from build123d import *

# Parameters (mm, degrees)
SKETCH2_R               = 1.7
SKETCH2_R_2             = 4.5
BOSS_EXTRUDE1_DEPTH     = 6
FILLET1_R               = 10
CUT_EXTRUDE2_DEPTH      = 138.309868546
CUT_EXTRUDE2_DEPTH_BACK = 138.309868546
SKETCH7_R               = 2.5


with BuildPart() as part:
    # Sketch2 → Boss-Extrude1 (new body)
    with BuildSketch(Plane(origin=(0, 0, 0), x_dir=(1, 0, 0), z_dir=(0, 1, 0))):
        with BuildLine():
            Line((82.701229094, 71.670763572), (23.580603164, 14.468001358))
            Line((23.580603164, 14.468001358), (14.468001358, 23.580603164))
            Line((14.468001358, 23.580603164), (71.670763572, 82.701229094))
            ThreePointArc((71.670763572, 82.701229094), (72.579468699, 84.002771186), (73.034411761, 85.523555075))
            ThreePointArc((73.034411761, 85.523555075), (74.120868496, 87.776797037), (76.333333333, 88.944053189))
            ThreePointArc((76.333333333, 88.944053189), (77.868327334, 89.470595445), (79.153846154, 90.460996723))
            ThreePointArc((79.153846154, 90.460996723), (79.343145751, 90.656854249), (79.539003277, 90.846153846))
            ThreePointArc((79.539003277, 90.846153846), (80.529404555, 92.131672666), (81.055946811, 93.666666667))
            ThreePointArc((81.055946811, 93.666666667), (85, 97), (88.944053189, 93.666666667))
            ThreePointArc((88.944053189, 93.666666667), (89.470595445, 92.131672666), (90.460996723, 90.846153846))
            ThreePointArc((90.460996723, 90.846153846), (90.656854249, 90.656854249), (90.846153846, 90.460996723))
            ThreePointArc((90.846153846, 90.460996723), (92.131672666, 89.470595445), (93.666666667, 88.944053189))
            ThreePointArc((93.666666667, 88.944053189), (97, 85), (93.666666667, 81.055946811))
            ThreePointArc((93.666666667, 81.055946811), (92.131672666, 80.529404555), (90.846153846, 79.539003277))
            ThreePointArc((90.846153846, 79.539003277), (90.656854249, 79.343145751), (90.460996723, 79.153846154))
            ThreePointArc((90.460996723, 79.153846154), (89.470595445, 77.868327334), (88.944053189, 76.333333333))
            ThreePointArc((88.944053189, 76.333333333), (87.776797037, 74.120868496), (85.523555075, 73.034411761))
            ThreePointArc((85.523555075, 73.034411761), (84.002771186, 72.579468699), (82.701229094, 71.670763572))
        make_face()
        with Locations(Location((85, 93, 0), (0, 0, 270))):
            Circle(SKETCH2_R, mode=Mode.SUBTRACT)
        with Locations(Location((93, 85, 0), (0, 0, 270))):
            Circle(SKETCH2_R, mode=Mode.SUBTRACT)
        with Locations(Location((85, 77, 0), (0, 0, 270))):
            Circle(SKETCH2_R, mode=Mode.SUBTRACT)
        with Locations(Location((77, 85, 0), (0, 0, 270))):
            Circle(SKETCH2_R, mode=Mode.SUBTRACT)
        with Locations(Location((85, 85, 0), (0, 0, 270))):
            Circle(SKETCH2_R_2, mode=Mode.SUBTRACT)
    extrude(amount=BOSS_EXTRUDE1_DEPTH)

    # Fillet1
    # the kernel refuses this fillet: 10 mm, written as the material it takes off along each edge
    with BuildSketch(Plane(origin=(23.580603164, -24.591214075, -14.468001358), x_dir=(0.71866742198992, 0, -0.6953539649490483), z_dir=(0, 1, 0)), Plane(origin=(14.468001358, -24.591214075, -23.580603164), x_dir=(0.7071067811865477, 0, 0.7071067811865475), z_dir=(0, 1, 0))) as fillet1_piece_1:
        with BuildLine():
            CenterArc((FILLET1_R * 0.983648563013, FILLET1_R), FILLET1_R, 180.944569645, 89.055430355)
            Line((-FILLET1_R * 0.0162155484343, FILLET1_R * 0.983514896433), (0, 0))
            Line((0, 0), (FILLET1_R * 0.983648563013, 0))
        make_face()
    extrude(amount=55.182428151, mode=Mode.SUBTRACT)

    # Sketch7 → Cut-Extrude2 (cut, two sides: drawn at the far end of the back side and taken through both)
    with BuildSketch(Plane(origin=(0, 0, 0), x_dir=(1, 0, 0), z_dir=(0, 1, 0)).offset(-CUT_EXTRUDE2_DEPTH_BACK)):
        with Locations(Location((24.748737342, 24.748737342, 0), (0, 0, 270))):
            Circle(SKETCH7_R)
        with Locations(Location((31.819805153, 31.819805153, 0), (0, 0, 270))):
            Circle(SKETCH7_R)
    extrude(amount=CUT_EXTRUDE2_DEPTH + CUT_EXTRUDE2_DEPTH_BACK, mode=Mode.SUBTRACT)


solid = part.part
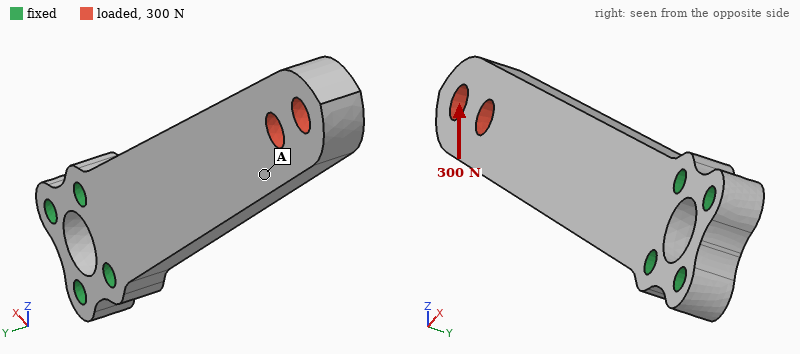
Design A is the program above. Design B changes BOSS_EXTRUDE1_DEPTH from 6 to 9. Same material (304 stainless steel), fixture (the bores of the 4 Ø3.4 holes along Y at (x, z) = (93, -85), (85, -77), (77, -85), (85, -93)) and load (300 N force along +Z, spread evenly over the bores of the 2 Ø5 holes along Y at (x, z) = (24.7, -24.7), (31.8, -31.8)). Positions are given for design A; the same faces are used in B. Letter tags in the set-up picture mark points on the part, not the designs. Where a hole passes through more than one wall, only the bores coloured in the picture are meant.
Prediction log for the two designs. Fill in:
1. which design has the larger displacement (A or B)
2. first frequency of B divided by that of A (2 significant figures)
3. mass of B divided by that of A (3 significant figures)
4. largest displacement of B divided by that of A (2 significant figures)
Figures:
A
1.5
1.50
0.67
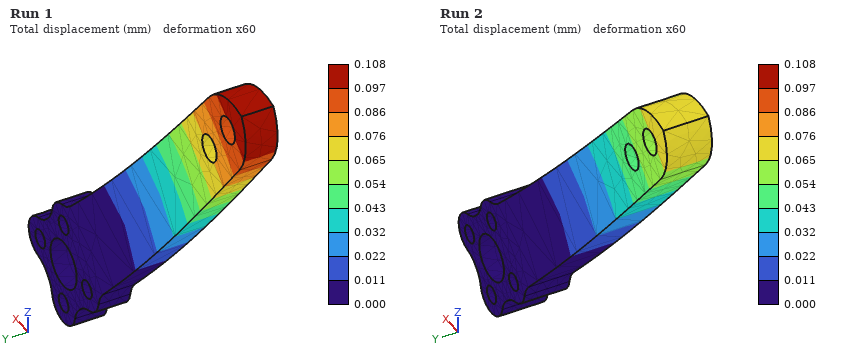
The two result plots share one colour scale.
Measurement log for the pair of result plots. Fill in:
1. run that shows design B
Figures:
Run 2
